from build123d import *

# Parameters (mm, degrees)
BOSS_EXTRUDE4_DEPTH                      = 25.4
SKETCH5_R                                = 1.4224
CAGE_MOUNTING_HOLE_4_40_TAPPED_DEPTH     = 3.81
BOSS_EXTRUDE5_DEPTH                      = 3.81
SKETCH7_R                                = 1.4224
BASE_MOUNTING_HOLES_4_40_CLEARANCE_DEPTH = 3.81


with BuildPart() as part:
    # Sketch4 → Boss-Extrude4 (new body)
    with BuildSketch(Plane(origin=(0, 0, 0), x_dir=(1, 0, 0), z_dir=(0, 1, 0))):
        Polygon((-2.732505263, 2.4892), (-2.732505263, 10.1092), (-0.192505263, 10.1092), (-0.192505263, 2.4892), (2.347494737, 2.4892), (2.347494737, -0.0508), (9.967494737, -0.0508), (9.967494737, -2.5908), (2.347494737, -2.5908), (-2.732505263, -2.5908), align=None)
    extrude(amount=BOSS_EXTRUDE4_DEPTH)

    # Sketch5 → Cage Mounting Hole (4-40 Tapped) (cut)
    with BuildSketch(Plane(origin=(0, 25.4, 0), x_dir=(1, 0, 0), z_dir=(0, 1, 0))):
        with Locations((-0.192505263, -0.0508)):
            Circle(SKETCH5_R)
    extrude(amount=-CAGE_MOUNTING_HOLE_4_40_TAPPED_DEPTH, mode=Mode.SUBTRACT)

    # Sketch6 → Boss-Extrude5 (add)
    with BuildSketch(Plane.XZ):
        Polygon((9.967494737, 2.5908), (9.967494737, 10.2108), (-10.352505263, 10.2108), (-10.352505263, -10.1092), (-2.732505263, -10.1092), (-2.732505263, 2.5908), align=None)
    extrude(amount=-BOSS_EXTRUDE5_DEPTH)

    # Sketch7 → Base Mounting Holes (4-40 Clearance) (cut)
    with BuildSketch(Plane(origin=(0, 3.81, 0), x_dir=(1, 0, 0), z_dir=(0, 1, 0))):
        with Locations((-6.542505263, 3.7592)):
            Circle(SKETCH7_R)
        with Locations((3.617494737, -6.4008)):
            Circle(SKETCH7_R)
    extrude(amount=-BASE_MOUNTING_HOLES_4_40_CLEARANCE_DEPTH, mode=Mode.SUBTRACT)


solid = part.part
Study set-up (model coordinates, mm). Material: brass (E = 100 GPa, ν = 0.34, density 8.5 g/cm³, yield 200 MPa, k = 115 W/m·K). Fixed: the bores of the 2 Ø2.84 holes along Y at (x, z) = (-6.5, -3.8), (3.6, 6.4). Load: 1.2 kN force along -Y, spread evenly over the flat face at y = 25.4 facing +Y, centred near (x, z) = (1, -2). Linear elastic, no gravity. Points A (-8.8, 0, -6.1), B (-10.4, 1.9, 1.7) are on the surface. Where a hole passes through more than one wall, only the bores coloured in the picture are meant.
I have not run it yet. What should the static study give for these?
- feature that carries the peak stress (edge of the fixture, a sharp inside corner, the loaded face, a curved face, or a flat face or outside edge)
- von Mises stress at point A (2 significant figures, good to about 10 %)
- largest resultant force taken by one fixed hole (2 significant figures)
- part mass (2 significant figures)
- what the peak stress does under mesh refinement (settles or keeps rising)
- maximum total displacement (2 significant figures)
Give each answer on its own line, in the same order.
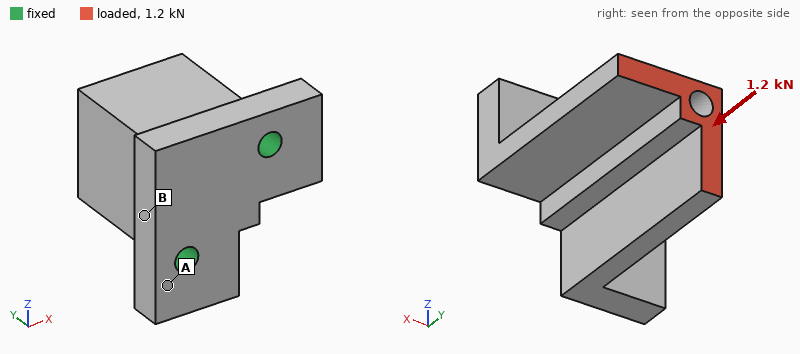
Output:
edge of the fixture
32 MPa
610 N
21 g
keeps rising
30 µm
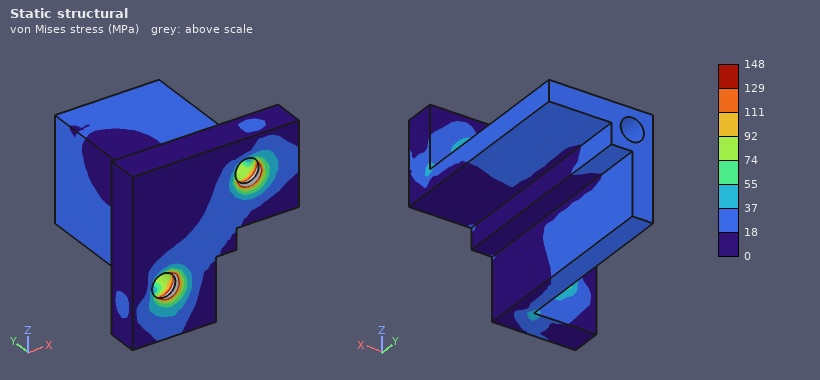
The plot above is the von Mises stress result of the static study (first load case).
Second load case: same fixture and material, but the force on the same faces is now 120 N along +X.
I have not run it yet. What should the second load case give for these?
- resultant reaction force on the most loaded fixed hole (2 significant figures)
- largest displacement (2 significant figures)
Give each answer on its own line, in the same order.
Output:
170 N
34 µm
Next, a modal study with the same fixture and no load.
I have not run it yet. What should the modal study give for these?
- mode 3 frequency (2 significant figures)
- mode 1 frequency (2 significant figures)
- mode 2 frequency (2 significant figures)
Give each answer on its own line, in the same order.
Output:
9100 Hz
4700 Hz
7000 Hz
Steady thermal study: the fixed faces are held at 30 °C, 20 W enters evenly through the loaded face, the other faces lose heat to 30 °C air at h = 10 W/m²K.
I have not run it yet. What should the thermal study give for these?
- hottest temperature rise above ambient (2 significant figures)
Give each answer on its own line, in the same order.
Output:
71 K
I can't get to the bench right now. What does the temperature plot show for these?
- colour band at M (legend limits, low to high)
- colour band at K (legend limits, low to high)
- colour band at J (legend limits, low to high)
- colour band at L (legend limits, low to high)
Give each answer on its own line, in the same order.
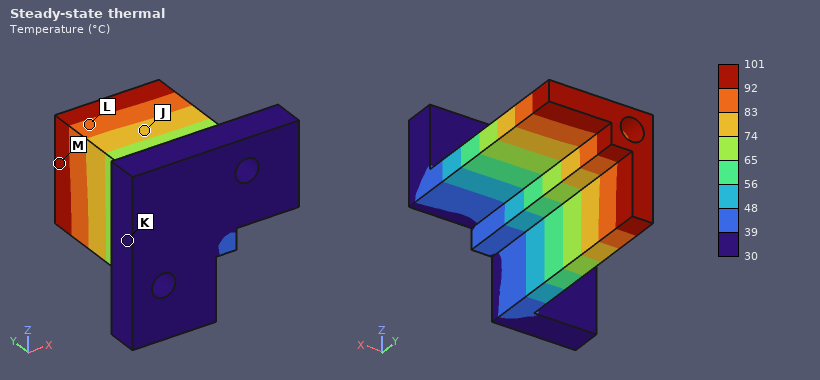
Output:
92 to 101 °C
30 to 39 °C
74 to 83 °C
83 to 92 °C
